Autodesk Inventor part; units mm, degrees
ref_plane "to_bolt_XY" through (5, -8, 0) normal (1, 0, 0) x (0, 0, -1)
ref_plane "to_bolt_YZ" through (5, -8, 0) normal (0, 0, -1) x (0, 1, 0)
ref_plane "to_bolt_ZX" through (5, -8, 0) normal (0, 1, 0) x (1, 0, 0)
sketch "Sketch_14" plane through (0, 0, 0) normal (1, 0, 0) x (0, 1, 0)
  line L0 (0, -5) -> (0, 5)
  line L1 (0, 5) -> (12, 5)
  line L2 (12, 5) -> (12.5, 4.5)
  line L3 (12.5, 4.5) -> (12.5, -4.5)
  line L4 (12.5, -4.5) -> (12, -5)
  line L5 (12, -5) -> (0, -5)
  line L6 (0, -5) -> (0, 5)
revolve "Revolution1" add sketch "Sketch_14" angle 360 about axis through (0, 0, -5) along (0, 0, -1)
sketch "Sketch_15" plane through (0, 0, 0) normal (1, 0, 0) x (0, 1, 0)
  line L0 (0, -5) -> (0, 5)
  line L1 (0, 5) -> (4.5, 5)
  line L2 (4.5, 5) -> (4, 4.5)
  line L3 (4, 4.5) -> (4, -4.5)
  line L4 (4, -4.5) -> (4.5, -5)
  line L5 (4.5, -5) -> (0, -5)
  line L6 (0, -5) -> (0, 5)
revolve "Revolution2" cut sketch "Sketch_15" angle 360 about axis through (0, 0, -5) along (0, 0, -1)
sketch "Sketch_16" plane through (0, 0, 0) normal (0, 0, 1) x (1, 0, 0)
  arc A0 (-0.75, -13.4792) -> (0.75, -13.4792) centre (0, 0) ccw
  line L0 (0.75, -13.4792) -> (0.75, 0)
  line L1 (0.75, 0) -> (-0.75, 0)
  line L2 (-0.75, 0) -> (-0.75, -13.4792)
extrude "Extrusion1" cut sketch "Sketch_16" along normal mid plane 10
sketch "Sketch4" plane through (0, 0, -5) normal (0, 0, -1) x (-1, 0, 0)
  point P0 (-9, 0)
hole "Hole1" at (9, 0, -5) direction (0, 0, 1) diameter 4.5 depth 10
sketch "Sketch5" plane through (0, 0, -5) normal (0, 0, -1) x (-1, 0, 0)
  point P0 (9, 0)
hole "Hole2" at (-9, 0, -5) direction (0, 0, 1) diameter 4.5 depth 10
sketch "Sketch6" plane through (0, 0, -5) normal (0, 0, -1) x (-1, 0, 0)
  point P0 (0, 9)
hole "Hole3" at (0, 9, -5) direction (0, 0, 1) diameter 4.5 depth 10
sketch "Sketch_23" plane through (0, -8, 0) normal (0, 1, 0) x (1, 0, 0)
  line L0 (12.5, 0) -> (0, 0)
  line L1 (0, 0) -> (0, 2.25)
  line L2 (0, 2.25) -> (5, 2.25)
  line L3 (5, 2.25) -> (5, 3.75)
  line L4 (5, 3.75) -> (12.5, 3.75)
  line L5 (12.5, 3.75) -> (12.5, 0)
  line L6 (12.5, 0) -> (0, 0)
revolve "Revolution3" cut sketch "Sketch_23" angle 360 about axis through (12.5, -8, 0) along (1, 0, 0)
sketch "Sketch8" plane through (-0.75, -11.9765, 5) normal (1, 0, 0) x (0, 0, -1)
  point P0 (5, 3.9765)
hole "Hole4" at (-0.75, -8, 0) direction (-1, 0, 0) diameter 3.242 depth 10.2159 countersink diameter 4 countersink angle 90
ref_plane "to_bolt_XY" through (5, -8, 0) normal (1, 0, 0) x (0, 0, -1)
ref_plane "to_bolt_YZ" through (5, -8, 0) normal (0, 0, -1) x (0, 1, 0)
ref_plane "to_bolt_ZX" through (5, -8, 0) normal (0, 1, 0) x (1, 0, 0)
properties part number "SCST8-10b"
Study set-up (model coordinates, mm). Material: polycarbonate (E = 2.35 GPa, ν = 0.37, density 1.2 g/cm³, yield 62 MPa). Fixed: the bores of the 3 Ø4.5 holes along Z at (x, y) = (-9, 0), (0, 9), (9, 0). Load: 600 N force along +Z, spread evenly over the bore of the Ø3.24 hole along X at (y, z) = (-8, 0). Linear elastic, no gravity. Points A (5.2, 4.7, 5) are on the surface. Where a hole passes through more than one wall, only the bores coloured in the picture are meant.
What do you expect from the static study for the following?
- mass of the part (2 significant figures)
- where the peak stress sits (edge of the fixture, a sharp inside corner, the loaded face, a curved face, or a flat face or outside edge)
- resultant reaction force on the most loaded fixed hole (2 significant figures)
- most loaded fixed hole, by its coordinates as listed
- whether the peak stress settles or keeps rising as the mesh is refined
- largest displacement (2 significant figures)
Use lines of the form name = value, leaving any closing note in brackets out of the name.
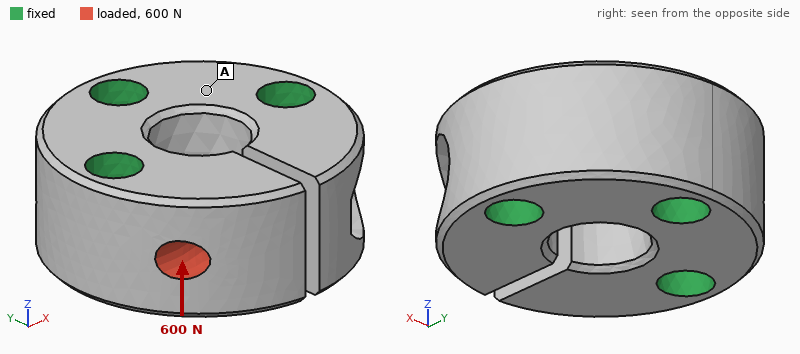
mass of the part = 4.1 g
where the peak stress sits = edge of the fixture
resultant reaction force on the most loaded fixed hole = 610 N
most loaded fixed hole, by its coordinates as listed = (-9, 0)
whether the peak stress settles or keeps rising as the mesh is refined = keeps rising
largest displacement = 0.22 mm
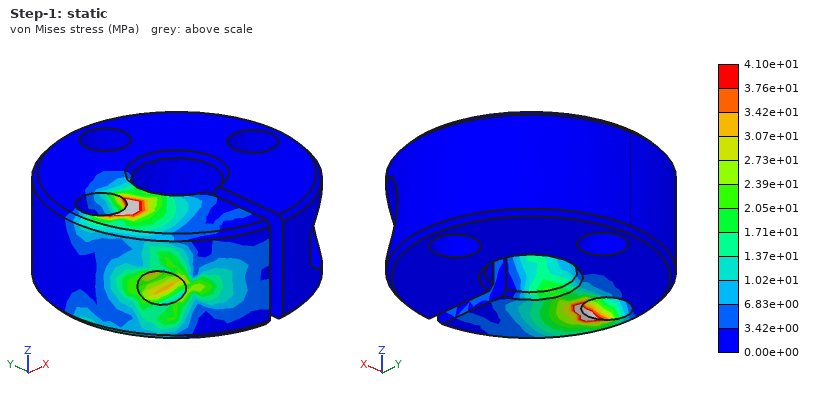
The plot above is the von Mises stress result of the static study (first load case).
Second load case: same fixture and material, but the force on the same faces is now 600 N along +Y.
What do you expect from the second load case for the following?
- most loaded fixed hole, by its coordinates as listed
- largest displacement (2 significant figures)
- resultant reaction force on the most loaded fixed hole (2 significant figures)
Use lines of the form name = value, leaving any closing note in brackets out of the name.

most loaded fixed hole, by its coordinates as listed = (-9, 0)
largest displacement = 0.14 mm
resultant reaction force on the most loaded fixed hole = 530 N
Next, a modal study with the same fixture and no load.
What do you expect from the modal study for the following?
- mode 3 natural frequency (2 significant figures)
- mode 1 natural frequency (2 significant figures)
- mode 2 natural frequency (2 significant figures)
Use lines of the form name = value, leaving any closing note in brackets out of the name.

mode 3 natural frequency = 10 kHz
mode 1 natural frequency = 9700 Hz
mode 2 natural frequency = 9800 Hz
